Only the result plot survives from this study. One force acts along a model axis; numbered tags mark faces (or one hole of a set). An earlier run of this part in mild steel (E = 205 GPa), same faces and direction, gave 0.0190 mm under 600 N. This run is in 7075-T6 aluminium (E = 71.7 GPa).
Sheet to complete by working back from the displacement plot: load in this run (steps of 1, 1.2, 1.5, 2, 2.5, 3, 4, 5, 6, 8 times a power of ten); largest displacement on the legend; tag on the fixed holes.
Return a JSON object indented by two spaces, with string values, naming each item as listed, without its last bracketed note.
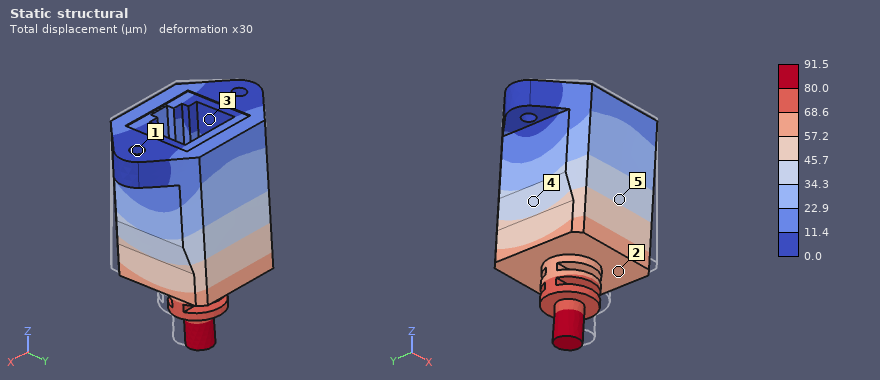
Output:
{
  "load in this run": "1 kN",
  "largest displacement on the legend": "91.5 µm",
  "tag on the fixed holes": "1"
}
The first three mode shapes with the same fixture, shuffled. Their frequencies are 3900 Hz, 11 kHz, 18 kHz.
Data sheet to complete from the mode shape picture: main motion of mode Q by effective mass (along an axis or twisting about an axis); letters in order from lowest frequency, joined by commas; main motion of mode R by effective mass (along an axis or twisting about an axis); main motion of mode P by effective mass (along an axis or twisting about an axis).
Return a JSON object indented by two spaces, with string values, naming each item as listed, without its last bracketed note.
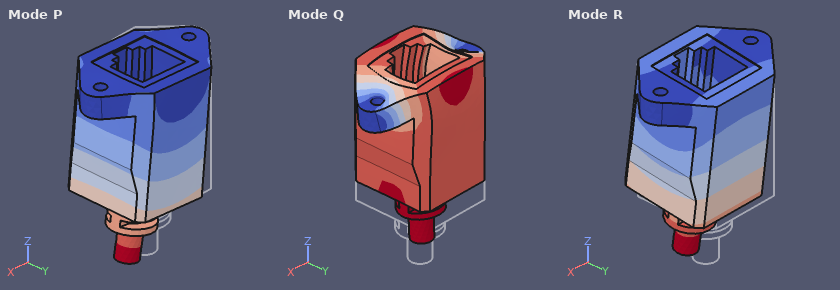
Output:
{
  "main motion of mode Q by effective mass": "along Z",
  "letters in order from lowest frequency, joined by commas": "R, P, Q",
  "main motion of mode R by effective mass": "along Y",
  "main motion of mode P by effective mass": "along X"
}
